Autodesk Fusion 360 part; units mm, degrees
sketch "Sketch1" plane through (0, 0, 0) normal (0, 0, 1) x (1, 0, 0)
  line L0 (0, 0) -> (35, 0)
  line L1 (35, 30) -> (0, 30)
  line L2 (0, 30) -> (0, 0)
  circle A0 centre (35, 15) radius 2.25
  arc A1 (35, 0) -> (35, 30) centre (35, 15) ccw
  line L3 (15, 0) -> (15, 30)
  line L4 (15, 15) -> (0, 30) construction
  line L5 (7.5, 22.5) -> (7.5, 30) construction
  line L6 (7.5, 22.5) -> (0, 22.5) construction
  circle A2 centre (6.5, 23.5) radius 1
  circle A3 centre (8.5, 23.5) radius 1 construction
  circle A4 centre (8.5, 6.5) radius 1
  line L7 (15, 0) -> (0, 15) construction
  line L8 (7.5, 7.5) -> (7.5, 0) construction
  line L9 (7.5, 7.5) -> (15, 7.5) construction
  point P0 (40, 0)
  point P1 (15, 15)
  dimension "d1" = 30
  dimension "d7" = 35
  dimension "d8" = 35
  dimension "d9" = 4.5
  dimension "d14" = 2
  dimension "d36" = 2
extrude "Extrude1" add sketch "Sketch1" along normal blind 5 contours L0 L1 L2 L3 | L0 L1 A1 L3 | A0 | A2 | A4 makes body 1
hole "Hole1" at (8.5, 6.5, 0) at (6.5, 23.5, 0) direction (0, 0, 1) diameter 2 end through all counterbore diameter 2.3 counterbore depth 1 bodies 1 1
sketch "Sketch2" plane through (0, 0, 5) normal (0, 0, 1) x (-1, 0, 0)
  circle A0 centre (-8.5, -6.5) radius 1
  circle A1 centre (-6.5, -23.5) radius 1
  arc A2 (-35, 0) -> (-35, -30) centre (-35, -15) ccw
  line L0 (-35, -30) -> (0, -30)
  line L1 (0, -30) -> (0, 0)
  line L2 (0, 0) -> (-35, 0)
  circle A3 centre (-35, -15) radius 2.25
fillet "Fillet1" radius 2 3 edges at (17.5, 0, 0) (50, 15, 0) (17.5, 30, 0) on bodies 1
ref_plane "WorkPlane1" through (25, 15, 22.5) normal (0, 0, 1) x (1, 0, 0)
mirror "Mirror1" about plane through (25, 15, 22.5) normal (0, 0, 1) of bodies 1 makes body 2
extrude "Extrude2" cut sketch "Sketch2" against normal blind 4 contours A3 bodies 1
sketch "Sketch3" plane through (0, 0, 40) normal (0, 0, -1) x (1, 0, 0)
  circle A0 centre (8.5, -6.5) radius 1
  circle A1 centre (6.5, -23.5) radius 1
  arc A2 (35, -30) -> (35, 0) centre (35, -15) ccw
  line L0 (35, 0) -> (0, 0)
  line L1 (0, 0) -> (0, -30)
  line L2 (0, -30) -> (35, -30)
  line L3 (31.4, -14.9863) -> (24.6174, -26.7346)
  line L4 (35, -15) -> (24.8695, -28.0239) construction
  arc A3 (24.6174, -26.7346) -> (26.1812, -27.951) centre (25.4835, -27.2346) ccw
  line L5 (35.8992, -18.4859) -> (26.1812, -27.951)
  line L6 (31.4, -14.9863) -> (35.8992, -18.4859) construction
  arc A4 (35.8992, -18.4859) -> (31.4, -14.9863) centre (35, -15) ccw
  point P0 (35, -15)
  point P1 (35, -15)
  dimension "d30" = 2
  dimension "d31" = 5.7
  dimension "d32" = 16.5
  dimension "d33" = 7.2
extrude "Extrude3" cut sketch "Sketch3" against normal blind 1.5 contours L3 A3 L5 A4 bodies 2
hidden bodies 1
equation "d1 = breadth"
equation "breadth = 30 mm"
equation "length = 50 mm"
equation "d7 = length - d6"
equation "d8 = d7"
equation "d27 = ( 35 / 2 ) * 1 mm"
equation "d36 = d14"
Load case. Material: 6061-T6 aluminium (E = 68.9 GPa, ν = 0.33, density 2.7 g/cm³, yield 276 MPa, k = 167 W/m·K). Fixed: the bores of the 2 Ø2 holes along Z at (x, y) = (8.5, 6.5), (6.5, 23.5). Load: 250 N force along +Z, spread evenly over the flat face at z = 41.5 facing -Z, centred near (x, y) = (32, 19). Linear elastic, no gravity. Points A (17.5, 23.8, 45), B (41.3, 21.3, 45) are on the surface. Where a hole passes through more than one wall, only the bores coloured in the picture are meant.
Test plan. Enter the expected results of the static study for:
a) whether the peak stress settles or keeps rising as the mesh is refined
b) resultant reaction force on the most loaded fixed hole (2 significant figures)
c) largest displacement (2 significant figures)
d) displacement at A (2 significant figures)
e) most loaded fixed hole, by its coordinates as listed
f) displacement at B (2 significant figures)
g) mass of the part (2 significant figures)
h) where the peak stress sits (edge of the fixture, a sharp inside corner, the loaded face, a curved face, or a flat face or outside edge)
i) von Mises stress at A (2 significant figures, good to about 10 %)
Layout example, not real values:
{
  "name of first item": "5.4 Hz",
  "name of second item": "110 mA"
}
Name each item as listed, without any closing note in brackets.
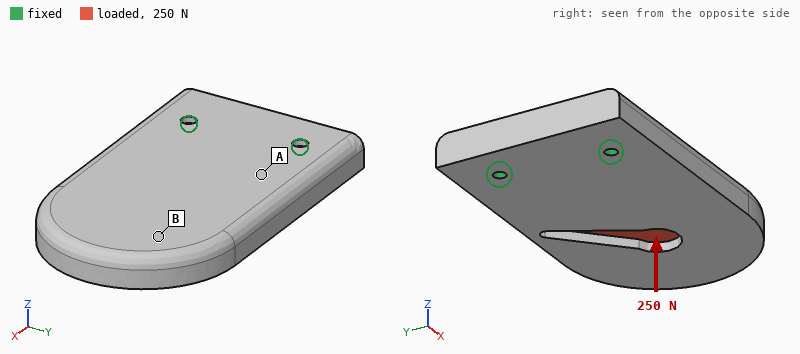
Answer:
{
  "whether the peak stress settles or keeps rising as the mesh is refined": "keeps rising",
  "resultant reaction force on the most loaded fixed hole": "140 N",
  "largest displacement": "0.17 mm",
  "displacement at A": "0.029 mm",
  "most loaded fixed hole, by its coordinates as listed": "(6.5, 23.5)",
  "displacement at B": "0.14 mm",
  "mass of the part": "18 g",
  "where the peak stress sits": "edge of the fixture",
  "von Mises stress at A": "29 MPa"
}
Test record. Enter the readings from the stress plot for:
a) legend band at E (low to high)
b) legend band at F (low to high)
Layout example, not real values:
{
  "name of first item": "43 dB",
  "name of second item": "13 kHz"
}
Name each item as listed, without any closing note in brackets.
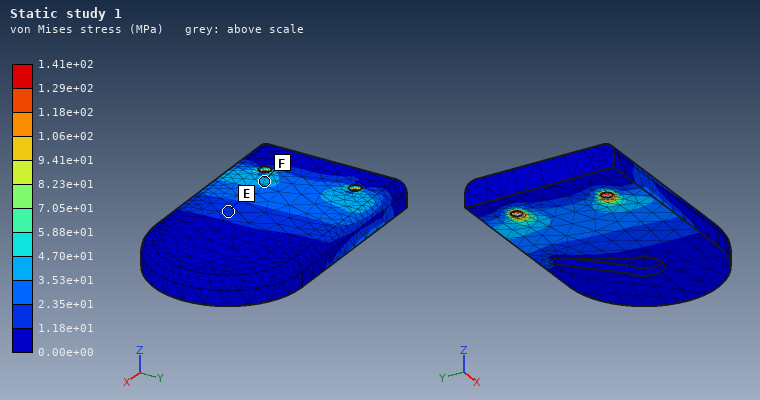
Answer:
{
  "legend band at E": "1.18e+01 to 2.35e+01 MPa",
  "legend band at F": "3.53e+01 to 4.70e+01 MPa"
}
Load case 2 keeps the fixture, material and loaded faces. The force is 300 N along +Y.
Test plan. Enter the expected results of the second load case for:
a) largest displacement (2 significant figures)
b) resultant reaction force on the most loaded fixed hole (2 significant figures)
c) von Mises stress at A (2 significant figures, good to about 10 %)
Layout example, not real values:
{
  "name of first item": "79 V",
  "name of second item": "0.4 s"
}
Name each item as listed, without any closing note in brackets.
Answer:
{
  "largest displacement": "10 µm",
  "resultant reaction force on the most loaded fixed hole": "450 N",
  "von Mises stress at A": "4.3 MPa"
}
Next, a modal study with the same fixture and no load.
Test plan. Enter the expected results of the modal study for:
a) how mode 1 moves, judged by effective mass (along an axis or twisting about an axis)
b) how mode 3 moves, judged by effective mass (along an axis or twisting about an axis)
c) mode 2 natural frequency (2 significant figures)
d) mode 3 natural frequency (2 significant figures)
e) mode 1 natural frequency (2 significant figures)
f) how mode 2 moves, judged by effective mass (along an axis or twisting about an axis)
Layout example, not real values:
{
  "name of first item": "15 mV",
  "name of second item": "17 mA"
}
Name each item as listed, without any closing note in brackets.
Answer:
{
  "how mode 1 moves, judged by effective mass": "along Z",
  "how mode 3 moves, judged by effective mass": "along Y",
  "mode 2 natural frequency": "7600 Hz",
  "mode 3 natural frequency": "9700 Hz",
  "mode 1 natural frequency": "2200 Hz",
  "how mode 2 moves, judged by effective mass": "twisting about X"
}
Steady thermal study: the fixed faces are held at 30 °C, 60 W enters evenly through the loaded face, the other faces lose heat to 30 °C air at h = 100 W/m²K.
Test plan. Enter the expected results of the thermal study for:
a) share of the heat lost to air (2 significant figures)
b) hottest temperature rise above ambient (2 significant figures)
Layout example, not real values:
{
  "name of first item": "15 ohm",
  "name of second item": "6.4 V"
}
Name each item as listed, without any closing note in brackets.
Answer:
{
  "share of the heat lost to air": "19 %",
  "hottest temperature rise above ambient": "67 K"
}
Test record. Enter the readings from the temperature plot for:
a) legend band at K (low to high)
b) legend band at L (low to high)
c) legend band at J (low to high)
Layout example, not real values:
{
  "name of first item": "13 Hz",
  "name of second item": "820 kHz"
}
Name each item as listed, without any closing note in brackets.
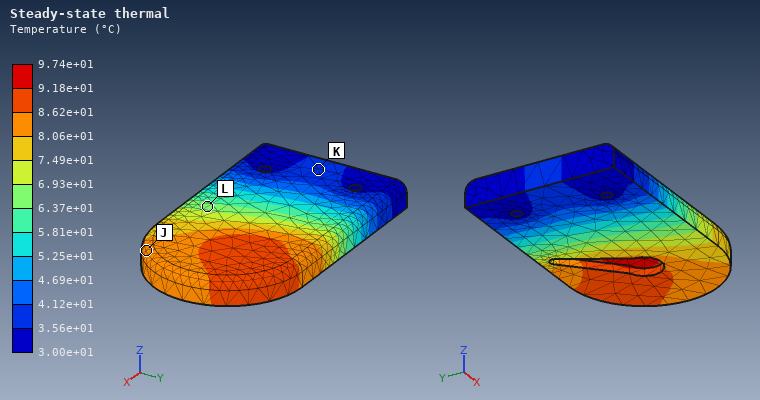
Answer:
{
  "legend band at K": "3.56e+01 to 4.12e+01 °C",
  "legend band at L": "6.37e+01 to 6.93e+01 °C",
  "legend band at J": "8.06e+01 to 8.62e+01 °C"
}
